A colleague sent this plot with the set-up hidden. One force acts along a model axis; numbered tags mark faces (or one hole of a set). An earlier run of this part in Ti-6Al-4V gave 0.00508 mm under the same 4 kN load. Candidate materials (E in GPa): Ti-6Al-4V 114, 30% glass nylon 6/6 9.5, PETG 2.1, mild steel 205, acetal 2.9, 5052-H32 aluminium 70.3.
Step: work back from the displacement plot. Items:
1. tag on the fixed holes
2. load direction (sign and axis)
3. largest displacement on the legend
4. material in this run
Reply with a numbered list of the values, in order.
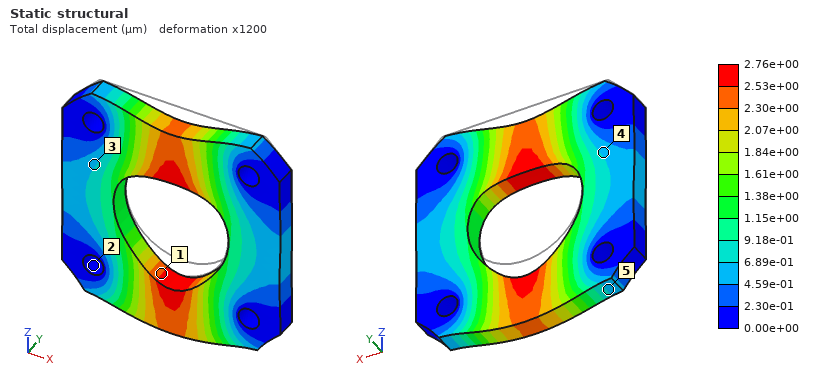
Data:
1. 2
2. -Z
3. 2.76e+00 µm
4. mild steel
